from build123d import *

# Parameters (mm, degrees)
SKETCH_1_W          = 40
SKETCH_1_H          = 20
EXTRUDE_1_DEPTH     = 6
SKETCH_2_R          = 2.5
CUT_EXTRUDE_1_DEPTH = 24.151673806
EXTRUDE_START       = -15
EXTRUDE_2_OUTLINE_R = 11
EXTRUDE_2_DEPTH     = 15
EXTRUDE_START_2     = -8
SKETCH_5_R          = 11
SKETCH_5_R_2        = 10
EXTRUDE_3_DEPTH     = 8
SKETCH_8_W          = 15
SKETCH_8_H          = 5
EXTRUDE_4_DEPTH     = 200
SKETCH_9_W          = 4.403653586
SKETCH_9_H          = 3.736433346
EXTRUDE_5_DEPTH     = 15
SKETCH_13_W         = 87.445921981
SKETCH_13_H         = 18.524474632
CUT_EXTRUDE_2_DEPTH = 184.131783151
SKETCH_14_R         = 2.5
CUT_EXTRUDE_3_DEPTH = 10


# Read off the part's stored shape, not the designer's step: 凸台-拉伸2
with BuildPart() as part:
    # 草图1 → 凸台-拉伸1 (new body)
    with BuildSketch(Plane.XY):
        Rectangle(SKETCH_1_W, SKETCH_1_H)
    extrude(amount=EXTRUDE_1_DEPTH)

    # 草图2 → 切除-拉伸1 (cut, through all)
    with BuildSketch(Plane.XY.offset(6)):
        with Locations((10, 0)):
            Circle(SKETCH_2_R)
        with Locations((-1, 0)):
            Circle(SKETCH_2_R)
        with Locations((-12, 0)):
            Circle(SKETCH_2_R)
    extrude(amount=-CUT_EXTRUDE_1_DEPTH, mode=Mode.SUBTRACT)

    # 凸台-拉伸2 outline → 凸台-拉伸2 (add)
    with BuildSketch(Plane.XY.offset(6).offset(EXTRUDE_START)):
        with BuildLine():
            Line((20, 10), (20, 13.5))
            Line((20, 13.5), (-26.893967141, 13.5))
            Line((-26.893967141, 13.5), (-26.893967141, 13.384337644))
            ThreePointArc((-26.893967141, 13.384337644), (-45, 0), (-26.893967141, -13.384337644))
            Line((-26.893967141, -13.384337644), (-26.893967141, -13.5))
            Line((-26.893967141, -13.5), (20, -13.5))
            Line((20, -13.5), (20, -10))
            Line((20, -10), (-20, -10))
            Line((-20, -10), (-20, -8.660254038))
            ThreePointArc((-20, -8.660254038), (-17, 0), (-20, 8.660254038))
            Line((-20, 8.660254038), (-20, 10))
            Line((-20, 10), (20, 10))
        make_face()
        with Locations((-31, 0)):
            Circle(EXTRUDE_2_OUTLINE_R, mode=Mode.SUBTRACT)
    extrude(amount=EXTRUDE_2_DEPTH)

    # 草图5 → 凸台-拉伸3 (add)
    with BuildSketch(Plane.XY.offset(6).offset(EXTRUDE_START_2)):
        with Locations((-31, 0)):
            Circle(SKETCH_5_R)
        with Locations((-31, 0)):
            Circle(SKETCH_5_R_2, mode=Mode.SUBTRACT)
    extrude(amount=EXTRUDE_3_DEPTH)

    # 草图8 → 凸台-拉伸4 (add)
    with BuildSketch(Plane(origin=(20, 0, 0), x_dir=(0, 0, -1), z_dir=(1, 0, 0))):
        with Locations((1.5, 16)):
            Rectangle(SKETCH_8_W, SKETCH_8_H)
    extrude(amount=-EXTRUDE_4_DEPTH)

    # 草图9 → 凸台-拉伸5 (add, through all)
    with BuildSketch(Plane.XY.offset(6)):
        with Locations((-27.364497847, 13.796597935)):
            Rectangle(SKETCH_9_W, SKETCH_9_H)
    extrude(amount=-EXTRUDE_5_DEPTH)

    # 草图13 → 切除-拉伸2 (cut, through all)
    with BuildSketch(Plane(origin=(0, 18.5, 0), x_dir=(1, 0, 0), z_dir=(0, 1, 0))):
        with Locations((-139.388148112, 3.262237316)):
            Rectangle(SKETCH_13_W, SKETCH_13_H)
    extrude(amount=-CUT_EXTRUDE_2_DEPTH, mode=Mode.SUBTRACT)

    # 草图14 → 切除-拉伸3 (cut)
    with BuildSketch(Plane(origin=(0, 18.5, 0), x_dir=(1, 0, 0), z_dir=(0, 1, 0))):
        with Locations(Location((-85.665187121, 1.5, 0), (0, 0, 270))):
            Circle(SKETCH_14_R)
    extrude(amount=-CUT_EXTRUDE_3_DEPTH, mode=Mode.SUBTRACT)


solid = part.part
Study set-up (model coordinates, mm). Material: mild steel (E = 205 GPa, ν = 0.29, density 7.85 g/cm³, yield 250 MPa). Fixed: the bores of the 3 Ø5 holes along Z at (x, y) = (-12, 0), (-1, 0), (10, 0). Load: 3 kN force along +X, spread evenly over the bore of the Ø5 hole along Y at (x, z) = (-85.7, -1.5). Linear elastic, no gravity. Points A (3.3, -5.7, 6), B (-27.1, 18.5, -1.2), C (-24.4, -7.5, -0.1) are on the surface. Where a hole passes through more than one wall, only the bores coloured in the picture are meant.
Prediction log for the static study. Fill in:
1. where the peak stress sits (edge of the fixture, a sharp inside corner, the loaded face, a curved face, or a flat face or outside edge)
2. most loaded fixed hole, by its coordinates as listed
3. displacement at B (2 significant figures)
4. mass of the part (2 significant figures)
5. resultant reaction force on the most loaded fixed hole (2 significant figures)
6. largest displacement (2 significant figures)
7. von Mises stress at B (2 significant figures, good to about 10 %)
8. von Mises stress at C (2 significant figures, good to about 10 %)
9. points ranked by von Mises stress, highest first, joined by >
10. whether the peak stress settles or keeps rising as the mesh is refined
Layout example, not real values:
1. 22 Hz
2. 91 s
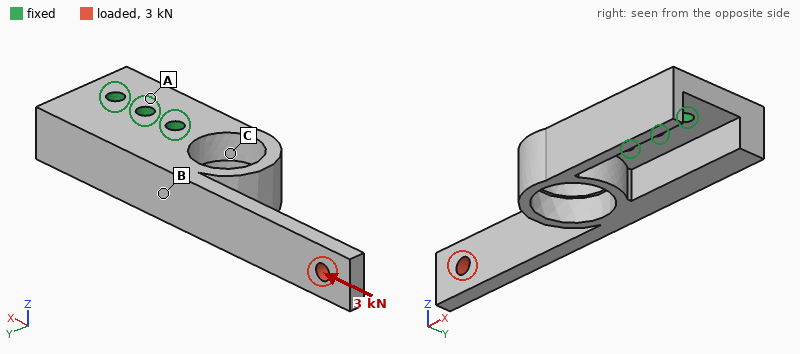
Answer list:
1. edge of the fixture
2. (-12, 0)
3. 10 µm
4. 170 g
5. 2.2 kN
6. 55 µm
7. 43 MPa
8. 17 MPa
9. B > C > A
10. keeps rising
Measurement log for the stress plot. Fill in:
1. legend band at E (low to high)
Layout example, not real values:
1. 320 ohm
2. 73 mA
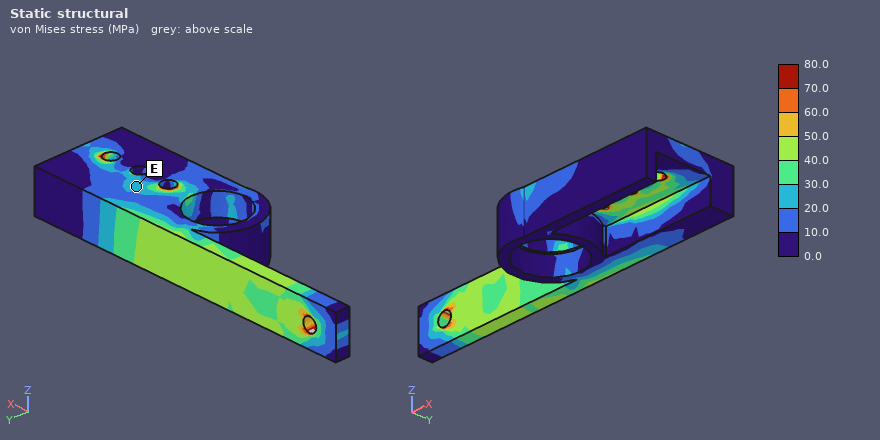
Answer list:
1. 20.0 to 30.0 MPa
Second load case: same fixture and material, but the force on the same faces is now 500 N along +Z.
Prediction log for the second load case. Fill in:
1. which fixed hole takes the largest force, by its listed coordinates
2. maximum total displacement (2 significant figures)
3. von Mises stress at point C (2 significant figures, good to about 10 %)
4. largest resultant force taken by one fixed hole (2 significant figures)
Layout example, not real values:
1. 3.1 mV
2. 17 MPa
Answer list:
1. (-12, 0)
2. 0.26 mm
3. 29 MPa
4. 1.8 kN
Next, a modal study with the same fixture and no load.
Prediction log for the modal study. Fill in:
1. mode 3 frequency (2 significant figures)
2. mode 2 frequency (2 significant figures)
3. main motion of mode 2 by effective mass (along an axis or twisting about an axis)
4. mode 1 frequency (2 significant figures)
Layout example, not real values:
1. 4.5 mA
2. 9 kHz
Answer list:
1. 5300 Hz
2. 1800 Hz
3. along Z
4. 980 Hz
